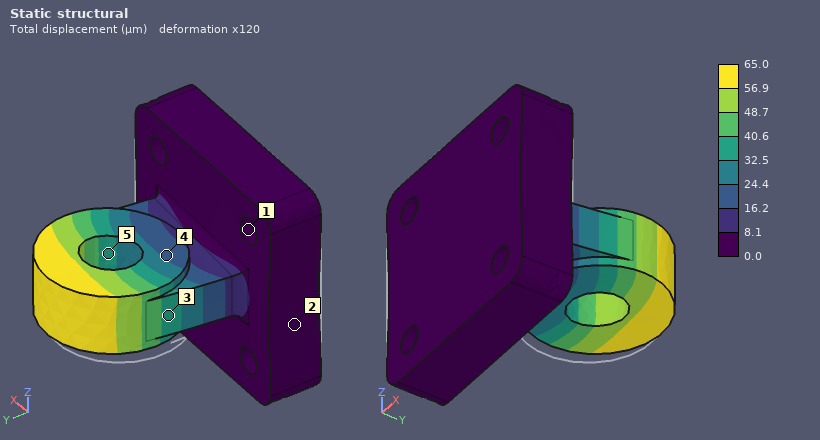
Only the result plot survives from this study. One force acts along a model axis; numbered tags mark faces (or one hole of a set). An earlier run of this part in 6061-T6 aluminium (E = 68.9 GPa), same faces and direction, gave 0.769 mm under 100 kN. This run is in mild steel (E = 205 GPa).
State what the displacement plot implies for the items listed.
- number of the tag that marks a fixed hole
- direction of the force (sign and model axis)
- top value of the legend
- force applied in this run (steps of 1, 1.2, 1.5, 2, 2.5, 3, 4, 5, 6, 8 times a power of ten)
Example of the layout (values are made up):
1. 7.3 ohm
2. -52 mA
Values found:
1. 1
2. +X
3. 65.0 µm
4. 25 kN
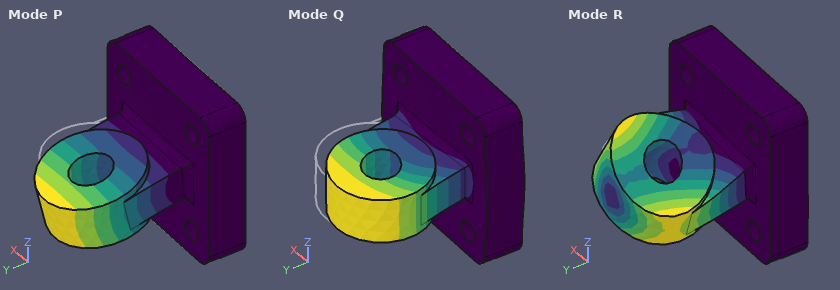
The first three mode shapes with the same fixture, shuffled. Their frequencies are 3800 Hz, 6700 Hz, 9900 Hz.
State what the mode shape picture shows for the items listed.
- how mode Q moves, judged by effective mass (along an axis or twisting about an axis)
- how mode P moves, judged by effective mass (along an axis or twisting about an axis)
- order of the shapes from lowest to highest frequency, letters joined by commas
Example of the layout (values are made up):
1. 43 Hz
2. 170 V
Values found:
1. along X
2. along Z
3. P, Q, R
